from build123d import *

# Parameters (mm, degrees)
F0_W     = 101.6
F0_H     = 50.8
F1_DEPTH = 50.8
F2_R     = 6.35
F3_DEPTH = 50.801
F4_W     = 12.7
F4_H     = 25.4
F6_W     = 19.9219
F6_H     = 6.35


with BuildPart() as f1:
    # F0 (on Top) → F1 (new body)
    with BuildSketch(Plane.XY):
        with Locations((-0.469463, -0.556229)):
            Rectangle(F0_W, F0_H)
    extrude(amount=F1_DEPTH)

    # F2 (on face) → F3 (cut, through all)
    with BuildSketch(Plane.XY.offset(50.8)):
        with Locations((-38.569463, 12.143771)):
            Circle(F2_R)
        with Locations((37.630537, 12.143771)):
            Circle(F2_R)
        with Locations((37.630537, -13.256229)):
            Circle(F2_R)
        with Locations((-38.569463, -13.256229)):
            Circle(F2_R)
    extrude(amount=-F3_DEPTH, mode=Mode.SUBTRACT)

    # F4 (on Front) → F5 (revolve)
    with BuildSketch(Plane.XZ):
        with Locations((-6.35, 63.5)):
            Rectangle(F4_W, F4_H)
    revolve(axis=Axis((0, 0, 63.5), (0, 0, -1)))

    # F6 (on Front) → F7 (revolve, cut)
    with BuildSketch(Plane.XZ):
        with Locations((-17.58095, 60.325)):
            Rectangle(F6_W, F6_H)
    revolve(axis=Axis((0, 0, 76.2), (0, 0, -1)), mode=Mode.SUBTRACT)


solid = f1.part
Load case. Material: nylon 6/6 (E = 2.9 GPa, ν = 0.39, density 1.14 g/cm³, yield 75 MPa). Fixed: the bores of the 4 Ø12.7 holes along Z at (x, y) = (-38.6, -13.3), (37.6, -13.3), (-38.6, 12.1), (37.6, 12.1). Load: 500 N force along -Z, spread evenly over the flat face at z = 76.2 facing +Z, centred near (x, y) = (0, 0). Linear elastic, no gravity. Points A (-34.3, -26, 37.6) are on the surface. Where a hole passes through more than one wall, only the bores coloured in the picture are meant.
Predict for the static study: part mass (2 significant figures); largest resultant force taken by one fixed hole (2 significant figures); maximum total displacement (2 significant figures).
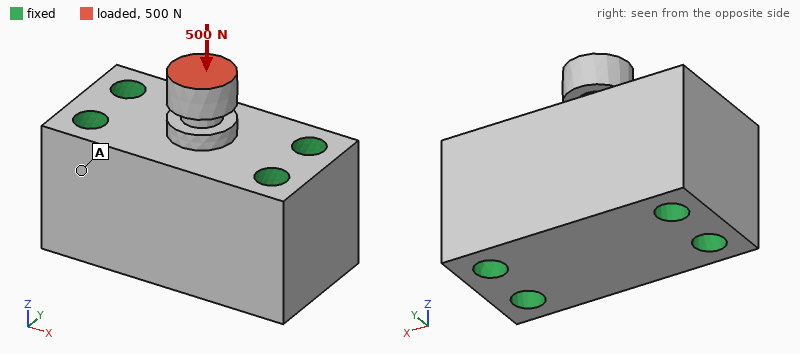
280 g
140 N
23 µm
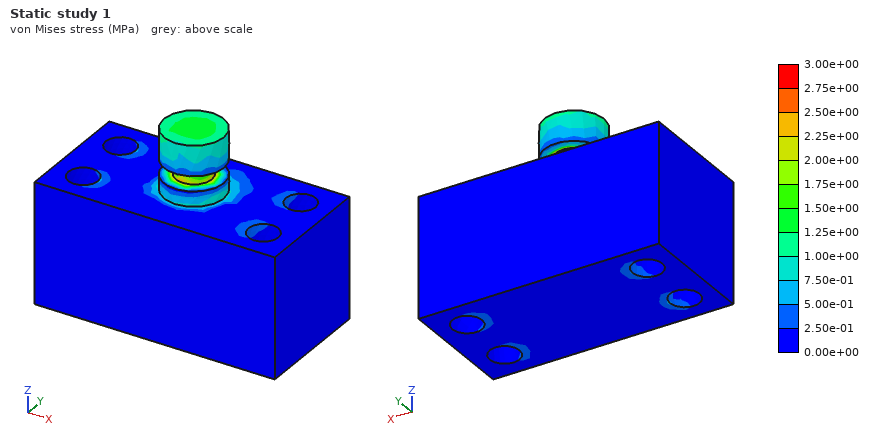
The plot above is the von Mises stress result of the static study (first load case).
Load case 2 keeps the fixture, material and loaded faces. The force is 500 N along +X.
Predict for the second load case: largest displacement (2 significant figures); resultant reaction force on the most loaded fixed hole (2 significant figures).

0.33 mm
220 N
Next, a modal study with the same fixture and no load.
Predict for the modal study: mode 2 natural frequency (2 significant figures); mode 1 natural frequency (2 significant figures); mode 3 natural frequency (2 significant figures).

3200 Hz
3000 Hz
4600 Hz
